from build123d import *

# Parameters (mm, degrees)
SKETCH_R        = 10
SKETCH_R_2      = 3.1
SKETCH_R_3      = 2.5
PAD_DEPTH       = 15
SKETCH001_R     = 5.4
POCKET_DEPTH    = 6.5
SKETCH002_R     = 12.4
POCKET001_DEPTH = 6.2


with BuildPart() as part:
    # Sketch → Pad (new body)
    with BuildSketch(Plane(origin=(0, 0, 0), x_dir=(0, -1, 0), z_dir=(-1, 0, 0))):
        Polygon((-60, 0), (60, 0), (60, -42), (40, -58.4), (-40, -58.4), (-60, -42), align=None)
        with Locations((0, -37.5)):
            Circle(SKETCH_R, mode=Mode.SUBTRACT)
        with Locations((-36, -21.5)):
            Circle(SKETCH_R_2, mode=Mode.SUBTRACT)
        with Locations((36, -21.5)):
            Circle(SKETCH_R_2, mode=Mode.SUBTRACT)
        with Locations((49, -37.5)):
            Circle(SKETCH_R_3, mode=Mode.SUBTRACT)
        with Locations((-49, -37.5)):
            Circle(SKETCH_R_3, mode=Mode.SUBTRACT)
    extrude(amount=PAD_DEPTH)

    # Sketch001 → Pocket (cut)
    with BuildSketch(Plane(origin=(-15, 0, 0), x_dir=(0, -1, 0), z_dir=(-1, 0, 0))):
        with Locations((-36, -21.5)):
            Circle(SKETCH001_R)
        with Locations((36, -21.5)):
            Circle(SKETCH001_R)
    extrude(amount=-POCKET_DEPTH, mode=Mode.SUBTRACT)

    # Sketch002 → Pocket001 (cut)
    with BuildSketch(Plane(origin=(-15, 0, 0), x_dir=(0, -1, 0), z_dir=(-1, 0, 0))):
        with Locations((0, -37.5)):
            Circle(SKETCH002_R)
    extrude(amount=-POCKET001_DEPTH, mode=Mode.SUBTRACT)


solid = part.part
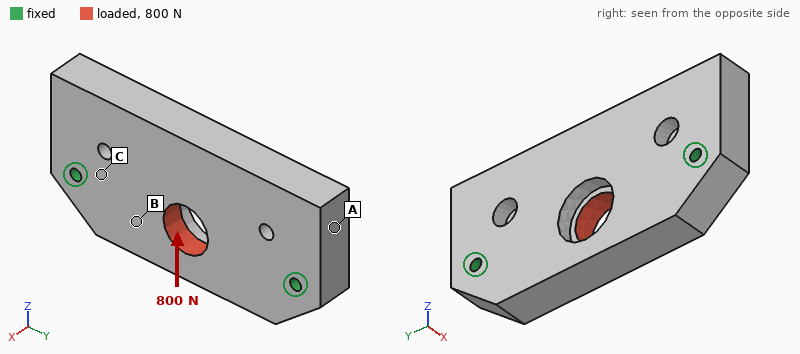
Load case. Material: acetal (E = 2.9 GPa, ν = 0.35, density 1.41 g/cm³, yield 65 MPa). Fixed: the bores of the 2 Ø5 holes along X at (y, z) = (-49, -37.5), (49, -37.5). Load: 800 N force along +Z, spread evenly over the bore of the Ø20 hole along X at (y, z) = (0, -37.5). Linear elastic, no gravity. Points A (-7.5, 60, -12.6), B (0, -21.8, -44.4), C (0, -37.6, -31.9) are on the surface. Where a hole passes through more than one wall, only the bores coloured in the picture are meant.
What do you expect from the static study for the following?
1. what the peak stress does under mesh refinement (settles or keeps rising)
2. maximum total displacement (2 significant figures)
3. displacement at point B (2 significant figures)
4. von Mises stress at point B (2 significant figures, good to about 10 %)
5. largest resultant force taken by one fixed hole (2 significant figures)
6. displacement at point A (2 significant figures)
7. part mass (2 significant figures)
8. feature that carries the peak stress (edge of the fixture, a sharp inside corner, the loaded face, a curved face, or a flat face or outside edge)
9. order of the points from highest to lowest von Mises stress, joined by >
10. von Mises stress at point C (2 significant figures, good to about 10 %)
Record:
keeps rising
69 µm
42 µm
1.3 MPa
410 N
15 µm
130 g
edge of the fixture
C > B > A
2.1 MPa
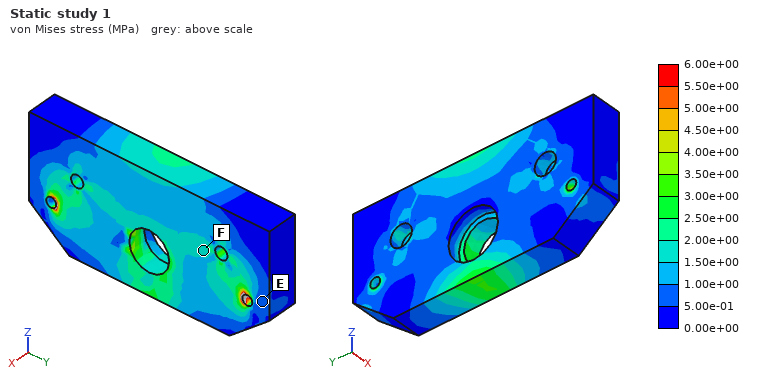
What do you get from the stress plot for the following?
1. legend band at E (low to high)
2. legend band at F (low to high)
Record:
5.00e-01 to 1.00e+00 MPa
1.50e+00 to 2.00e+00 MPa
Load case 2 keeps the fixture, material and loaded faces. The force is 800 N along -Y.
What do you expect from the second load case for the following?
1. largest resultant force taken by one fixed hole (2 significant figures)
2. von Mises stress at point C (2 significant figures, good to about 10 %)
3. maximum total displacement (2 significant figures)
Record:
400 N
1.2 MPa
19 µm
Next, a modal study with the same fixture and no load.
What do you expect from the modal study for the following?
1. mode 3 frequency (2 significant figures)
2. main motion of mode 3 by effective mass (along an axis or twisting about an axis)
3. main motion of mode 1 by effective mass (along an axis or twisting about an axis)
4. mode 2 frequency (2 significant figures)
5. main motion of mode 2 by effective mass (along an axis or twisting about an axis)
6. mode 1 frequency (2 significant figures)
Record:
2200 Hz
twisting about Z
along X
1800 Hz
along X
1100 Hz
